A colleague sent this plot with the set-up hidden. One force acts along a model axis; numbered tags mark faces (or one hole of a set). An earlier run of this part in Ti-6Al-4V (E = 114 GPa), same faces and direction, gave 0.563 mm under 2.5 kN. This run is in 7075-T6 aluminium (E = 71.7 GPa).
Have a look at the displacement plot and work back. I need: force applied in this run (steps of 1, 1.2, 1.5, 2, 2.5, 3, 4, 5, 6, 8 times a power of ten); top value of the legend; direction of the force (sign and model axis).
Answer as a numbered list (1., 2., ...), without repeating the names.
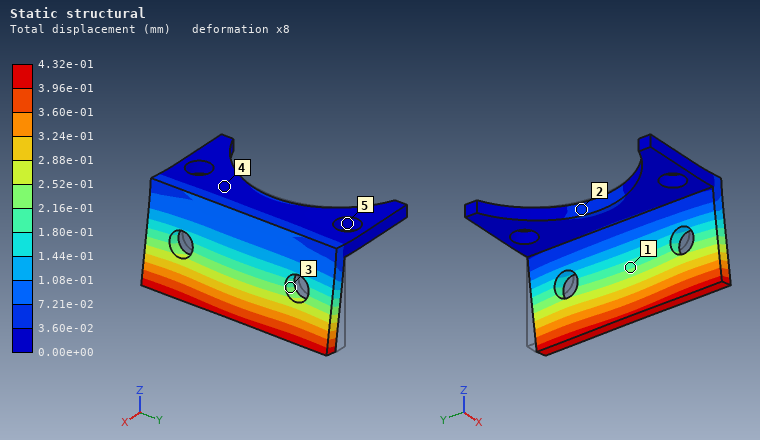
1. 1.2 kN
2. 4.32e-01 mm
3. +X
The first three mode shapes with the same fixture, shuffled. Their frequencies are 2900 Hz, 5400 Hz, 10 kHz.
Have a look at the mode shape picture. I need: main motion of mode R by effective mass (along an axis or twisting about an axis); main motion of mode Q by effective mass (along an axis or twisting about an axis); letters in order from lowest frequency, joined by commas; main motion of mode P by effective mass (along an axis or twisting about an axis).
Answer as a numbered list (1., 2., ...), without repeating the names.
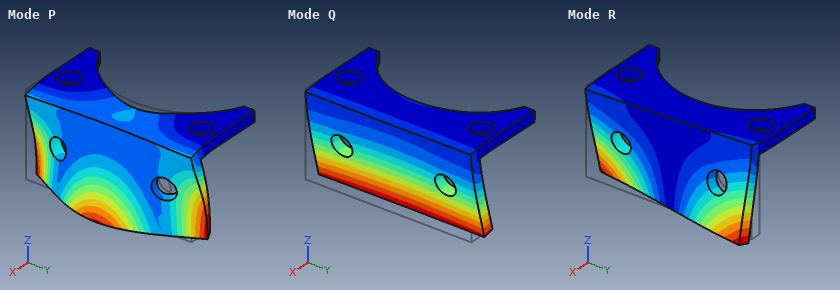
1. twisting about Z
2. along X
3. Q, R, P
4. along Z
